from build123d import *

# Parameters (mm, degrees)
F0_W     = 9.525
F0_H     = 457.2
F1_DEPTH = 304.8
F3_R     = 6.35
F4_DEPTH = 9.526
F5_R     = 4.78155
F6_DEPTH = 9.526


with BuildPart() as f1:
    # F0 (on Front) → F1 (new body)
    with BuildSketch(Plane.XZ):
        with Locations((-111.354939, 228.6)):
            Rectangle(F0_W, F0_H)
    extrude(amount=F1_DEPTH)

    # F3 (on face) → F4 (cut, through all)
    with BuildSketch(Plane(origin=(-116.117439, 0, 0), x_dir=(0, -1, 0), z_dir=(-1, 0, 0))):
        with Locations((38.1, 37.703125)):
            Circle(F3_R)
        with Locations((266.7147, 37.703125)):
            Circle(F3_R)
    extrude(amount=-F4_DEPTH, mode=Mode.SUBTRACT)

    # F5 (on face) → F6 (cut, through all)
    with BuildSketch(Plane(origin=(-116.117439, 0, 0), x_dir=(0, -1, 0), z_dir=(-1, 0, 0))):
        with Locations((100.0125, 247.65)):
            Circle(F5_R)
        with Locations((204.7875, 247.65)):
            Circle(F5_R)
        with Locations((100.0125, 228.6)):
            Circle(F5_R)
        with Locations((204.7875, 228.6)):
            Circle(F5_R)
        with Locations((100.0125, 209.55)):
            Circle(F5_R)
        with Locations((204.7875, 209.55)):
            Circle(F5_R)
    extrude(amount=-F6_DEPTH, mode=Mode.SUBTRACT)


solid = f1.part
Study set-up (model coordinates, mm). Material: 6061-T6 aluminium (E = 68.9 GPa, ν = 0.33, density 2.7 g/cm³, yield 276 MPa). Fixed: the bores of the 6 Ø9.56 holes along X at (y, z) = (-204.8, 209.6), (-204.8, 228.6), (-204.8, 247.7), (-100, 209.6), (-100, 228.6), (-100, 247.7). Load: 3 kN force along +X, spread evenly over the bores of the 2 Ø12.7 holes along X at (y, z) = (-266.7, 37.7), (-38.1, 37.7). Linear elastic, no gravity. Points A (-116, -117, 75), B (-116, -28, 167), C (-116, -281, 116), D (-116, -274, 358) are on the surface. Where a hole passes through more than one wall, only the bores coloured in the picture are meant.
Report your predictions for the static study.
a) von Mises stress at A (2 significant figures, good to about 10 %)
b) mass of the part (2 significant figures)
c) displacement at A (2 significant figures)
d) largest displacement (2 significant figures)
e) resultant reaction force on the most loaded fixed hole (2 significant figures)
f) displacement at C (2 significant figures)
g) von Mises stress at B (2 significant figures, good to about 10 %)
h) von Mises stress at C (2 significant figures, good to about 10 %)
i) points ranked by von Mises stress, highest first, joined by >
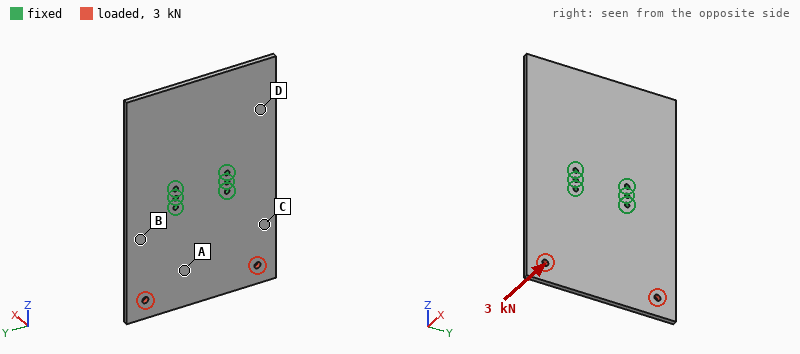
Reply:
26 MPa
3.6 kg
2.5 mm
5.1 mm
6.1 kN
1.6 mm
70 MPa
49 MPa
B > C > A > D
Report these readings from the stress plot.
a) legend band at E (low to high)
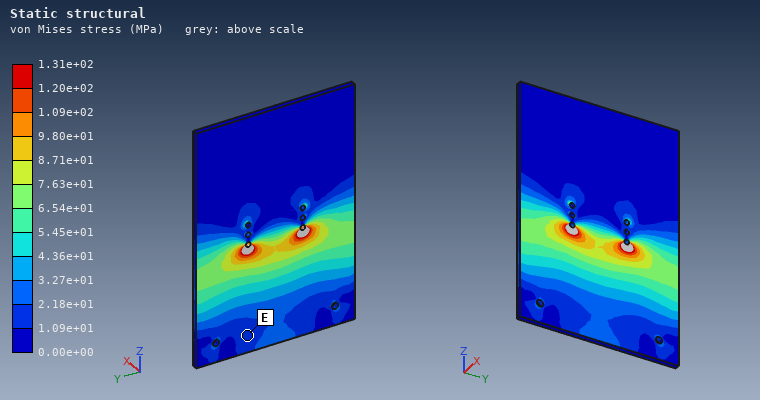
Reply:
1.09e+01 to 2.18e+01 MPa
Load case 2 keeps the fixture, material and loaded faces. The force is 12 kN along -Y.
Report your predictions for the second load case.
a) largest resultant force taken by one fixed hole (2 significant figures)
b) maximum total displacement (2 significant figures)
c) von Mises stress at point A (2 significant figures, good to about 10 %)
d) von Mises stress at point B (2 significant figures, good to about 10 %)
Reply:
11 kN
0.13 mm
9.7 MPa
6.9 MPa
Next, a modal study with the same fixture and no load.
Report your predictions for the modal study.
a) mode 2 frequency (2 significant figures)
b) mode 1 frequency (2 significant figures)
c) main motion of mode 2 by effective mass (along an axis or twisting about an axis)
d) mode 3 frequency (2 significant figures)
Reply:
170 Hz
160 Hz
along X
270 Hz
